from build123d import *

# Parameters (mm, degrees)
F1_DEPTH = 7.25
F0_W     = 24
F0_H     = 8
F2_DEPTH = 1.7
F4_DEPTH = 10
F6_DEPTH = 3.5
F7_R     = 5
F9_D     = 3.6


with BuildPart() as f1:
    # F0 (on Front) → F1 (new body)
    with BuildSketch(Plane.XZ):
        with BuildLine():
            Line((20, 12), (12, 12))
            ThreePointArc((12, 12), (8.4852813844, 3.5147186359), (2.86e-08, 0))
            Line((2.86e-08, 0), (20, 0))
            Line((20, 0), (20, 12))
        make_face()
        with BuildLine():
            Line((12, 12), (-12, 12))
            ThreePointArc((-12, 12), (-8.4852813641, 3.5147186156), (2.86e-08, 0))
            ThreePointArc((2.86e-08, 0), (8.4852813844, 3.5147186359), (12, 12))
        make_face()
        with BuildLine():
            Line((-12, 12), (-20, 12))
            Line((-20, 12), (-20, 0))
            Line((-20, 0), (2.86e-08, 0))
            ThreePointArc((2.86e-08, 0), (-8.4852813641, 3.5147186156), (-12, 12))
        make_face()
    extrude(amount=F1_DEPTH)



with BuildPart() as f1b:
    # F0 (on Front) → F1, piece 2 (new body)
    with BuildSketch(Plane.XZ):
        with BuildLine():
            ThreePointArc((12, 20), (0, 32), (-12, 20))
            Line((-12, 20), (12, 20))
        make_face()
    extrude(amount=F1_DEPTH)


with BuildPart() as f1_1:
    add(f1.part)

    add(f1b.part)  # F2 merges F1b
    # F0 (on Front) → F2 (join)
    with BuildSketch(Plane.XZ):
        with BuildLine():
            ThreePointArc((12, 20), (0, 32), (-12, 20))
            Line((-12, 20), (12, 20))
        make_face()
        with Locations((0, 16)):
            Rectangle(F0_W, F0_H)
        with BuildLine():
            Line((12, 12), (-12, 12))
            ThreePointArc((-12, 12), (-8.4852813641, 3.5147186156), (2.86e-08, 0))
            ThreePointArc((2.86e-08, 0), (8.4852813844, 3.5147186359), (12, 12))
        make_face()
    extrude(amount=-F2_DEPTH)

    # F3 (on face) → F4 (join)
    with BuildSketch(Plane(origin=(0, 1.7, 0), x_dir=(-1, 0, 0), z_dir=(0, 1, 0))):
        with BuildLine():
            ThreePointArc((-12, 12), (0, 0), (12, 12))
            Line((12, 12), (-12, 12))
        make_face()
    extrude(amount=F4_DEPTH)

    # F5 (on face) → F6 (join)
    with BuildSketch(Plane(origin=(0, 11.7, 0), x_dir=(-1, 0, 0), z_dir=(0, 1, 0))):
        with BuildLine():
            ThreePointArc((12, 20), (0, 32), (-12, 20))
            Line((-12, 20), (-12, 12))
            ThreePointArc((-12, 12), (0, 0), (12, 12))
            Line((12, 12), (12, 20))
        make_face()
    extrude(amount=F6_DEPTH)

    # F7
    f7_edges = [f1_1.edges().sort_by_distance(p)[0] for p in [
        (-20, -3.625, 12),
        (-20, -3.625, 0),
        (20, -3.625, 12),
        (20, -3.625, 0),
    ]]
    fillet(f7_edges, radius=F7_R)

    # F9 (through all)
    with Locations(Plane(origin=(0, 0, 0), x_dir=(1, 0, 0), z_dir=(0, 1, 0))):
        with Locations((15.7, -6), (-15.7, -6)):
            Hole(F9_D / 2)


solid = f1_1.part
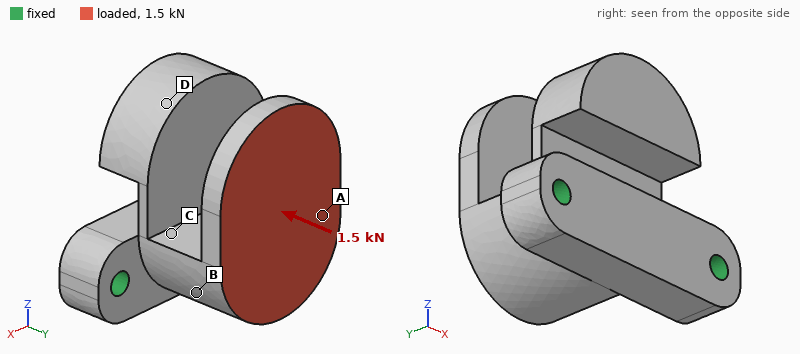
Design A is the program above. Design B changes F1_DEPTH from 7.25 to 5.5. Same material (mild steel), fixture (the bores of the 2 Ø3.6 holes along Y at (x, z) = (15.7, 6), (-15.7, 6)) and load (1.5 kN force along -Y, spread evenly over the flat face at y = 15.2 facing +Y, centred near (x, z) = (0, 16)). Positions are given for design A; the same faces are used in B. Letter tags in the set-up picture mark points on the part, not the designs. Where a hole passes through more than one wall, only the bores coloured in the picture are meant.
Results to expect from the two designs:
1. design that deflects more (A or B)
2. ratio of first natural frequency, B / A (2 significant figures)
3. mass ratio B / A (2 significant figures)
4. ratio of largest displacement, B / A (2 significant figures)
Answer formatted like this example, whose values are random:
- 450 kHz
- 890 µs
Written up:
- B
- 1.1
- 0.89
- 1.2
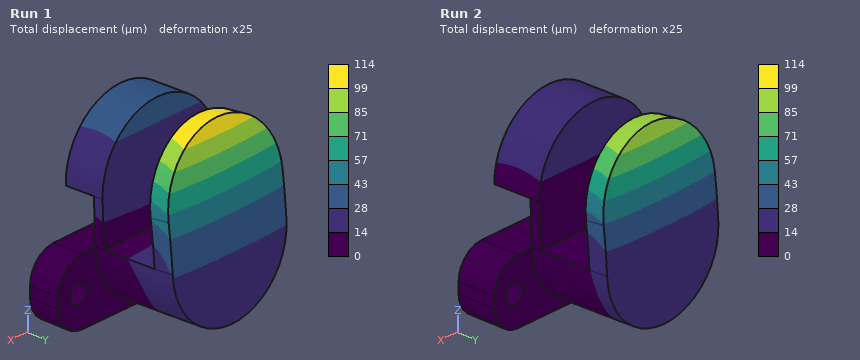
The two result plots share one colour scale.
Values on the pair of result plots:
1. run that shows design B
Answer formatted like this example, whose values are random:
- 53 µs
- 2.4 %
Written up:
- Run 1
